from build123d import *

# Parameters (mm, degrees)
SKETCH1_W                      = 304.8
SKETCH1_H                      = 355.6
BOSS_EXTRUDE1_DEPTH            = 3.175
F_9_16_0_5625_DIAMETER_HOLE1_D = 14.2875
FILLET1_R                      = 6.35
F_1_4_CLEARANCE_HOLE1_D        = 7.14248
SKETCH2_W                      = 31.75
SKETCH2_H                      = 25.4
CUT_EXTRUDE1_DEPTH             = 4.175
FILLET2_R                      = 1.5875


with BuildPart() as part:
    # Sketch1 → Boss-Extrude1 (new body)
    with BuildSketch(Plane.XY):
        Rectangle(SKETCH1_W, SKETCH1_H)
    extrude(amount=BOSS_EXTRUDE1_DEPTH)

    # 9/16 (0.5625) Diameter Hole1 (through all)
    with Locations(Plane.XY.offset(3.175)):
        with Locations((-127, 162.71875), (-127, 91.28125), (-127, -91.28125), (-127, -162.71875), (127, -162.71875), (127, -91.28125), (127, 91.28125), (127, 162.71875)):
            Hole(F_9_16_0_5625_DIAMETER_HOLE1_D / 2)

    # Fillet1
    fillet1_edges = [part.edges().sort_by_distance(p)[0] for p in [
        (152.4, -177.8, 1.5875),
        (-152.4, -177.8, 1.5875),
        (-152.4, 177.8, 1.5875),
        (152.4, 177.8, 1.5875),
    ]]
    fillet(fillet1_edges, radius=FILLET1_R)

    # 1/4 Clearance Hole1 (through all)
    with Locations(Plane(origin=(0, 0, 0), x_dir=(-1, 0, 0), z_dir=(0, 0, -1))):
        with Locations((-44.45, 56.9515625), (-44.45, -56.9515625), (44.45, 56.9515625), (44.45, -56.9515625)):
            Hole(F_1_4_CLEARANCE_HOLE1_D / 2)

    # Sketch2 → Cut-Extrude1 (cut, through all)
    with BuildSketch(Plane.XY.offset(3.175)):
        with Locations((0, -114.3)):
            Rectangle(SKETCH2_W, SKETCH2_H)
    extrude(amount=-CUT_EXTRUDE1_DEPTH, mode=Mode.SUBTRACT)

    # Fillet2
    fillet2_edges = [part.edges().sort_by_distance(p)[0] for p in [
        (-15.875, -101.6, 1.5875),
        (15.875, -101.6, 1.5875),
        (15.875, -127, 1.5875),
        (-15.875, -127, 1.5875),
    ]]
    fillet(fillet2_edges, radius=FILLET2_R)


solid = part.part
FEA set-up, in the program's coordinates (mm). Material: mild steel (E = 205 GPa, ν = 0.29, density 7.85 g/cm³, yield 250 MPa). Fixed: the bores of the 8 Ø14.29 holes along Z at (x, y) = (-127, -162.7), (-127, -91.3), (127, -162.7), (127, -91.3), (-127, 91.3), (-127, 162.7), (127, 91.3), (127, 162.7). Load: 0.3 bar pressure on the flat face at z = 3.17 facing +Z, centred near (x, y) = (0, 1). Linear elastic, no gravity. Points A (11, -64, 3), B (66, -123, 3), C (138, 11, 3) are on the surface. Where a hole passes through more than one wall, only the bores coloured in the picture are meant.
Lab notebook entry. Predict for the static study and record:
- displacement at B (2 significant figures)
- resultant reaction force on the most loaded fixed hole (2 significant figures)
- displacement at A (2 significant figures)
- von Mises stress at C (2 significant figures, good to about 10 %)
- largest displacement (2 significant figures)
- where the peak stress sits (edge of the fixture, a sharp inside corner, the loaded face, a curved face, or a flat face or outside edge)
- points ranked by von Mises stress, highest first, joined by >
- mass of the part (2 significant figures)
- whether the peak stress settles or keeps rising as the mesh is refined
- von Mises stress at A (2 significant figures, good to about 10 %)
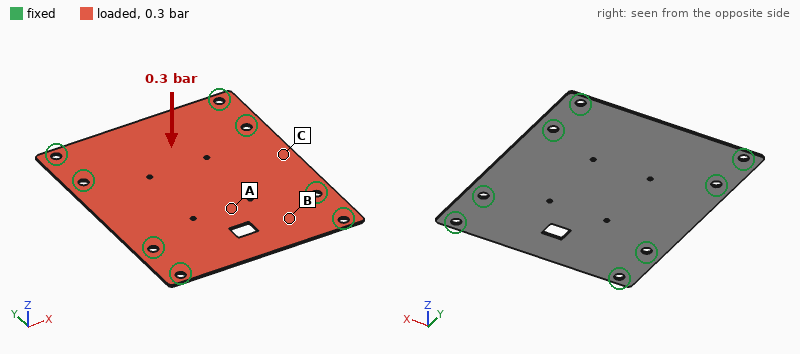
0.31 mm
600 N
0.72 mm
28 MPa
0.81 mm
edge of the fixture
A > C > B
2.6 kg
keeps rising
47 MPa
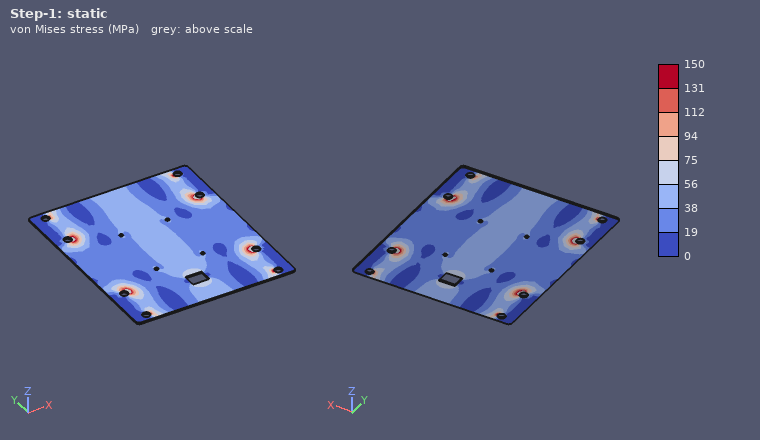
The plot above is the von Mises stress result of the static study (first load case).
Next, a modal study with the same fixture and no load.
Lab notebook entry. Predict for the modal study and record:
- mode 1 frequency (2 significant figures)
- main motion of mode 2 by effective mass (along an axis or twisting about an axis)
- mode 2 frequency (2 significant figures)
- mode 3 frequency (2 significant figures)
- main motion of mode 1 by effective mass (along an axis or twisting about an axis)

240 Hz
twisting about X
300 Hz
370 Hz
along Z
